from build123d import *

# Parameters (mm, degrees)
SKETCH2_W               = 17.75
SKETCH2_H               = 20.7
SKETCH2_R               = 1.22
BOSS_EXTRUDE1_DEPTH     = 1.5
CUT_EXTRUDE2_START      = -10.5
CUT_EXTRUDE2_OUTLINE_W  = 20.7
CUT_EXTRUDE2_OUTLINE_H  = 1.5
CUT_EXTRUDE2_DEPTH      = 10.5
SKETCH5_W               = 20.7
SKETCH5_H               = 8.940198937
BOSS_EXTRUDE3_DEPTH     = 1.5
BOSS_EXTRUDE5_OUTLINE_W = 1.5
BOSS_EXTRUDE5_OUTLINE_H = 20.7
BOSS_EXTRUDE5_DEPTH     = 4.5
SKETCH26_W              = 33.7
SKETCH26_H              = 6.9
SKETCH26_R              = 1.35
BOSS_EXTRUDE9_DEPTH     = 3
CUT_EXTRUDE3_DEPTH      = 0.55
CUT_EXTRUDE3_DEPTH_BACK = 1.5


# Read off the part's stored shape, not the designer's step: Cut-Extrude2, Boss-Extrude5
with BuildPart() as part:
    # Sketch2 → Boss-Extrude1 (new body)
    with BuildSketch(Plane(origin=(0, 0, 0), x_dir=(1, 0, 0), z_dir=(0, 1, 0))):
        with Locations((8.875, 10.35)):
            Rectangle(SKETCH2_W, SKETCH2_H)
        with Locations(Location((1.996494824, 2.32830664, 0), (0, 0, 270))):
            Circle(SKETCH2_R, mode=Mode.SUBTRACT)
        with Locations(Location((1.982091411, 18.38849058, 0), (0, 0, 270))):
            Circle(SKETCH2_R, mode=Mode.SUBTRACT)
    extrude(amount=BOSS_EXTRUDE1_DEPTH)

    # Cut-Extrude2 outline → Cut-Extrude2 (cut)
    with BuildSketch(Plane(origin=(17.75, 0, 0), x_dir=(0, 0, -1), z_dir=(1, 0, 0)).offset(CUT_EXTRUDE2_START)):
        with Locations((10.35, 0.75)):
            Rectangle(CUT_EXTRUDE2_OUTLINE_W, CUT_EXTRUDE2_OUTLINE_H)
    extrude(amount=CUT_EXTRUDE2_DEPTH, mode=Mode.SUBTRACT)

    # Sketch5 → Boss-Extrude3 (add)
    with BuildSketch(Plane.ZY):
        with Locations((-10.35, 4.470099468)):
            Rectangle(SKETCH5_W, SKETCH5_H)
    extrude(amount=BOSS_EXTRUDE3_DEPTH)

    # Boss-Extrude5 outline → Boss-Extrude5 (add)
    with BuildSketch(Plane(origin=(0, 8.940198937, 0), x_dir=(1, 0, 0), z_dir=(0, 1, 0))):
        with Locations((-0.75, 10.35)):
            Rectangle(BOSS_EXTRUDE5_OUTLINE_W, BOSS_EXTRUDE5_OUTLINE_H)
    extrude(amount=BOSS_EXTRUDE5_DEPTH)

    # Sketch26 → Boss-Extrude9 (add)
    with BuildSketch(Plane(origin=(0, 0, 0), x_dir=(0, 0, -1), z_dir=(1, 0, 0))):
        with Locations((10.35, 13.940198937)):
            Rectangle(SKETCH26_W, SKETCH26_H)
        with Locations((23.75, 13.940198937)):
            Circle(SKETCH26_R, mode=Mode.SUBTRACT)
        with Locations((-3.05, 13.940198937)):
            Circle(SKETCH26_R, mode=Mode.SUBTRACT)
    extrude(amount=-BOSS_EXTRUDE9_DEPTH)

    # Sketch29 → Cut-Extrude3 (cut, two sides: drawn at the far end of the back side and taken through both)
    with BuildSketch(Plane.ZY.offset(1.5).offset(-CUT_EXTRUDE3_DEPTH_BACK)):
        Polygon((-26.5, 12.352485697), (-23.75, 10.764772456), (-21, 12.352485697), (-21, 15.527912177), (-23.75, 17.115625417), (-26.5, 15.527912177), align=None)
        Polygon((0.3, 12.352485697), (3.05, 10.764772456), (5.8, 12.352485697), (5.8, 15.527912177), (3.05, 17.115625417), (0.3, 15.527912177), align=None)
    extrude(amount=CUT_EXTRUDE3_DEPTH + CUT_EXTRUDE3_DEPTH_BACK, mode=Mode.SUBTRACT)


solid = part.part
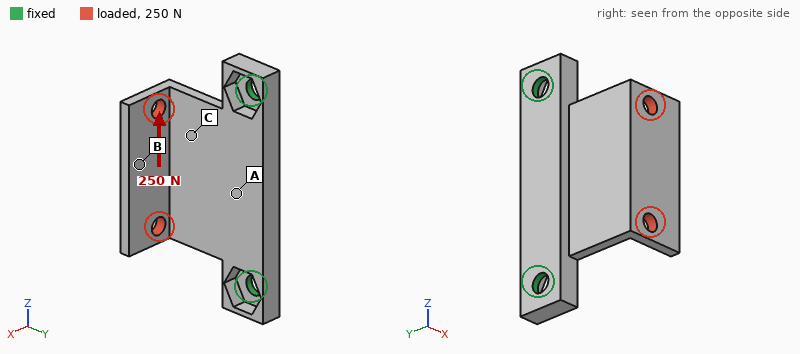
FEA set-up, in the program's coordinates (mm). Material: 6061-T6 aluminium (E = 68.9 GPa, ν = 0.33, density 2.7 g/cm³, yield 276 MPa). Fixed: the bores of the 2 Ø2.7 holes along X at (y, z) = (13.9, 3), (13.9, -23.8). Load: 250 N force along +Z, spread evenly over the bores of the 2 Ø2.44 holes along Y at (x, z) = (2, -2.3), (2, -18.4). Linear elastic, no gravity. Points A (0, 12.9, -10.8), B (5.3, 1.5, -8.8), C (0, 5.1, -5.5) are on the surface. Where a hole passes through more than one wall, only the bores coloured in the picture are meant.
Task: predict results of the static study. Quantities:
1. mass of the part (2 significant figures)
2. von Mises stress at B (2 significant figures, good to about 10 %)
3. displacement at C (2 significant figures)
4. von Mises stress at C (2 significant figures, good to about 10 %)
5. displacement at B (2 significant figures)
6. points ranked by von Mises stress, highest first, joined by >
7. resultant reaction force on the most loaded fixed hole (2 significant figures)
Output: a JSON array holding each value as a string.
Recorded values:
["3.0 g", "17 MPa", "15 µm", "56 MPa", "42 µm", "C > B > A", "190 N"]
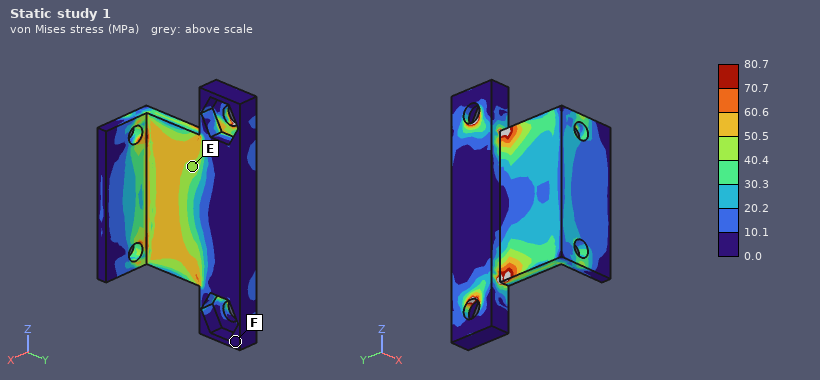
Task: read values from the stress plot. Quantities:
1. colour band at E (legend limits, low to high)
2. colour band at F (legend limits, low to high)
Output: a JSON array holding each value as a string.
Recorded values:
["40.4 to 50.5 MPa", "0.0 to 10.1 MPa"]
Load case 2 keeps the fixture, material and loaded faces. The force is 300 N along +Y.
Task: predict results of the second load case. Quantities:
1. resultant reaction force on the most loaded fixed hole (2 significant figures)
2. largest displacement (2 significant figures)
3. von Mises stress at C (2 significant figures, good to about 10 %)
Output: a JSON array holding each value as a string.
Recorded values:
["150 N", "0.38 mm", "100 MPa"]
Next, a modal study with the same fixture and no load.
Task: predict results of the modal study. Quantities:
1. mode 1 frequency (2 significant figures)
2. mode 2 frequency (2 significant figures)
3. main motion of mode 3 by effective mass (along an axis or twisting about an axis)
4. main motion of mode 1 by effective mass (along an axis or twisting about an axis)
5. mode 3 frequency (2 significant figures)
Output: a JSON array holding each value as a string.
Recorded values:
["3200 Hz", "7700 Hz", "along X", "along X", "11 kHz"]
